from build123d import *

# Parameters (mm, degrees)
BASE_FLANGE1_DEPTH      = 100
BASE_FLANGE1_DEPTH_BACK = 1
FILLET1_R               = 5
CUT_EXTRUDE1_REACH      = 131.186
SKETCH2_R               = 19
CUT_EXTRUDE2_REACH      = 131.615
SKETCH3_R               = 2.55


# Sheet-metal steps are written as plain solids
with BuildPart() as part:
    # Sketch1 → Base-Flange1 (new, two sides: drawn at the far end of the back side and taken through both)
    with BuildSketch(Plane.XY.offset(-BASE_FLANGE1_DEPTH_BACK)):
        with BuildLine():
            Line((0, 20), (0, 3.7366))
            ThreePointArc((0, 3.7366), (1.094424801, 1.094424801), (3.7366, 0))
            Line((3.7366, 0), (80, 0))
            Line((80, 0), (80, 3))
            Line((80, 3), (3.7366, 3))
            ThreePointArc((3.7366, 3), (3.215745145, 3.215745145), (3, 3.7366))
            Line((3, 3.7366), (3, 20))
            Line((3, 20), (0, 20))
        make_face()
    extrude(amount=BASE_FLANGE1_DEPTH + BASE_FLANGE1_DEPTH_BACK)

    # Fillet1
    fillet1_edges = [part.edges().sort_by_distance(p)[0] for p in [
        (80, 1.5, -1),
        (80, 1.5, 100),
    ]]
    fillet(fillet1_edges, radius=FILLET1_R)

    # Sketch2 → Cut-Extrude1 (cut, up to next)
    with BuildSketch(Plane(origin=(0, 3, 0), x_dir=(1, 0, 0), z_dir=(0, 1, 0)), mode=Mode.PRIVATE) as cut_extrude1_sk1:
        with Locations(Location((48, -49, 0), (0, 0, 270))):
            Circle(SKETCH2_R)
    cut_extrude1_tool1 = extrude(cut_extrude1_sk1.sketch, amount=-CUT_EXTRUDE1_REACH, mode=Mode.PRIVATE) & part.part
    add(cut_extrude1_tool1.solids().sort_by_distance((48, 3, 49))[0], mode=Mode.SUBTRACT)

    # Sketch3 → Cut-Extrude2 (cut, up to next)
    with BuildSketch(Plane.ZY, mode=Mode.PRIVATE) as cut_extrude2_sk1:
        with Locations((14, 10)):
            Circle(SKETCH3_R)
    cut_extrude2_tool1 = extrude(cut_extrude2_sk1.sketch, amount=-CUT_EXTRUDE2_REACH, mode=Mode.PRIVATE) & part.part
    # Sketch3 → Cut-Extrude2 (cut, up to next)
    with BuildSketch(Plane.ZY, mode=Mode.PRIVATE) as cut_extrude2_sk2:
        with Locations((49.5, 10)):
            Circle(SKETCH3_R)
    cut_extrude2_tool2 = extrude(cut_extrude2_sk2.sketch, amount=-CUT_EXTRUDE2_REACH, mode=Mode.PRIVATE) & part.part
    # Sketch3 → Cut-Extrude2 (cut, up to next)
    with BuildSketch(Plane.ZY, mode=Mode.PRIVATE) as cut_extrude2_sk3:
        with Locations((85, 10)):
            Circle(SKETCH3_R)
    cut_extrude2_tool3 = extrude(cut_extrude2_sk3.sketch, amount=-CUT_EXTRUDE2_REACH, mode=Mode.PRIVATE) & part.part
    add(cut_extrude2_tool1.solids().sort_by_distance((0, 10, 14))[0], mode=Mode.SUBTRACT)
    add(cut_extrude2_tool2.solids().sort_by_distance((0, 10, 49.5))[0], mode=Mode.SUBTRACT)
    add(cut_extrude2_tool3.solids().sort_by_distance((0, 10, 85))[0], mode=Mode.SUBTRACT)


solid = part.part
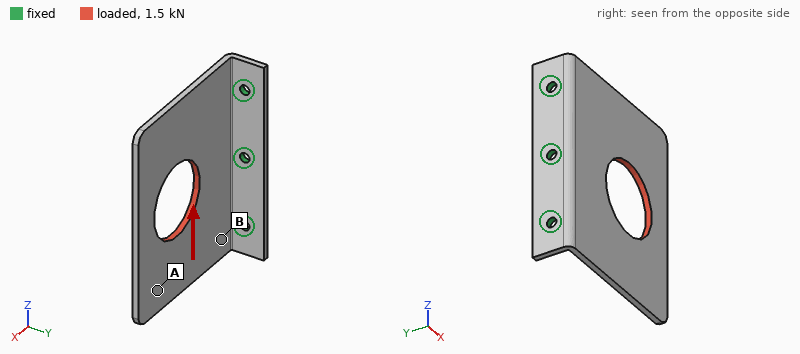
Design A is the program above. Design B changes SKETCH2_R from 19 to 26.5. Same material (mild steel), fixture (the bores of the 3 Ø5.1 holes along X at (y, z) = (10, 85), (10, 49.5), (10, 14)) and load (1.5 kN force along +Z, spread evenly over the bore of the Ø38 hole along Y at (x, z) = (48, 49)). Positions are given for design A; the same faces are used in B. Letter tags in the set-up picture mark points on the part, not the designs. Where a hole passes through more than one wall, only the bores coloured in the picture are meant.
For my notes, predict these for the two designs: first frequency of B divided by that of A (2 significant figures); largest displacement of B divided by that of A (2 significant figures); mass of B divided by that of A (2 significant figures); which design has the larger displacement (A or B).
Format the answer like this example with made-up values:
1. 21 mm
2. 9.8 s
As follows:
1. 1.0
2. 1.2
3. 0.87
4. B
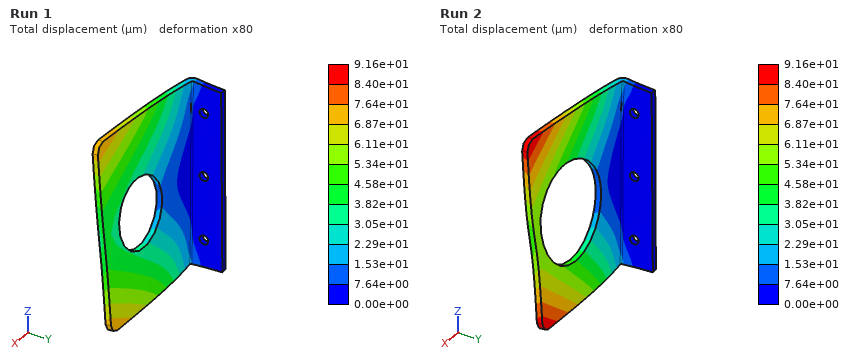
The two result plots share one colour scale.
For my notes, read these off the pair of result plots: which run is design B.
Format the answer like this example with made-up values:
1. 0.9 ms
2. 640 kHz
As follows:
1. Run 2
